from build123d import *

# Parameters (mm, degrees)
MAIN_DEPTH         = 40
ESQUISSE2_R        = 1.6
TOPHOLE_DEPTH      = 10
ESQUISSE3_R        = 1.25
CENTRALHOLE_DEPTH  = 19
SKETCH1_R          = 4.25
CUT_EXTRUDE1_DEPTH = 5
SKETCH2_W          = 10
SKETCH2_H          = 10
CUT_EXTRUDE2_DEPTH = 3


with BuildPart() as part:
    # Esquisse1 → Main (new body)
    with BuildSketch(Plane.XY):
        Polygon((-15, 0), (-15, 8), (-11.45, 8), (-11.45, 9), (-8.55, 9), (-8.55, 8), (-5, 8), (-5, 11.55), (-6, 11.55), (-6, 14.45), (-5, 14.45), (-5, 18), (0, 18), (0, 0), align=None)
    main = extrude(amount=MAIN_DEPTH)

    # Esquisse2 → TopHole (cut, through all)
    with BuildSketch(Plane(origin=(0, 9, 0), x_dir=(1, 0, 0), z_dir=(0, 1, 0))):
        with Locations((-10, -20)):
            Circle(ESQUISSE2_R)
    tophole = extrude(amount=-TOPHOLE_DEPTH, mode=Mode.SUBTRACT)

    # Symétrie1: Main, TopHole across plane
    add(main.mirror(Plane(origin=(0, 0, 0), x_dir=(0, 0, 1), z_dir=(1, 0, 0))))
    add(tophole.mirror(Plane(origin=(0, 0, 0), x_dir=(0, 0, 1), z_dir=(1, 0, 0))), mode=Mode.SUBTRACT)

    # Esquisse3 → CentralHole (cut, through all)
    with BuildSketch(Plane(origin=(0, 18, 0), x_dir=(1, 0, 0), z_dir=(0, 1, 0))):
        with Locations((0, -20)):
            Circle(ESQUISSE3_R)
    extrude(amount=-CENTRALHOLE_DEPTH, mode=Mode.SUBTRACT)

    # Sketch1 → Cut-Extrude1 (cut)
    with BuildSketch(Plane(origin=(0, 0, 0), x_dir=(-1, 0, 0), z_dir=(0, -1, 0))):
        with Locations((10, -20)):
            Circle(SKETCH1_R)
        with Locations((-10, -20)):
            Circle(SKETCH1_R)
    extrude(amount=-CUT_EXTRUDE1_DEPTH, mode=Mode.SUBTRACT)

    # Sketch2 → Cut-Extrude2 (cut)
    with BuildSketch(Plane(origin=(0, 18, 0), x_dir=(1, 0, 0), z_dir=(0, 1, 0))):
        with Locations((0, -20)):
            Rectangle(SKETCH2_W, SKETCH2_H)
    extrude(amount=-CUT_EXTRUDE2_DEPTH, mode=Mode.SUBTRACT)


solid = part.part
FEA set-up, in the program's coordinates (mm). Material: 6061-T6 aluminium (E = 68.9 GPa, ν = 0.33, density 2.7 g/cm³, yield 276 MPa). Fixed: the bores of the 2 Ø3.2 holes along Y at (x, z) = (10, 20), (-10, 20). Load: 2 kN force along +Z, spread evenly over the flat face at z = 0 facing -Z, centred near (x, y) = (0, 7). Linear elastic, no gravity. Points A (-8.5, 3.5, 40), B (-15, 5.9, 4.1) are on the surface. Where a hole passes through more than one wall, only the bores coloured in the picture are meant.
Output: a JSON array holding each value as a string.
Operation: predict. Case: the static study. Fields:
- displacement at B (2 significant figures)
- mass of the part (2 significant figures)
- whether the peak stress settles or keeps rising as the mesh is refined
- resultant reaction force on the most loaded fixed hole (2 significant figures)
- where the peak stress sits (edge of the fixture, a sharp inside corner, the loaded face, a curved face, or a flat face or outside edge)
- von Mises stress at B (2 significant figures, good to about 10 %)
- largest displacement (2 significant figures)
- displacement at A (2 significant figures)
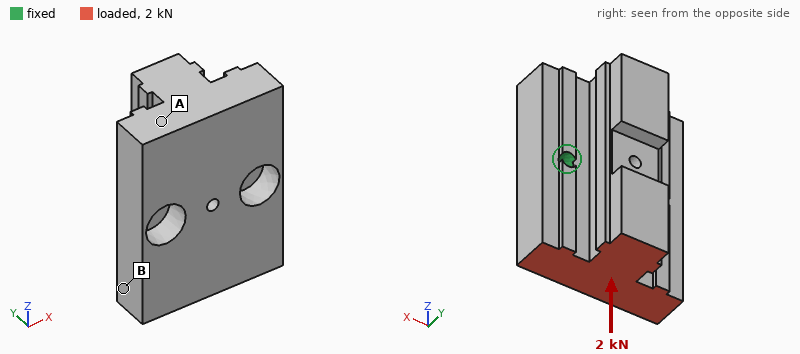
["3.0 µm", "35 g", "keeps rising", "1.0 kN", "edge of the fixture", "6.2 MPa", "4.2 µm", "1.5 µm"]
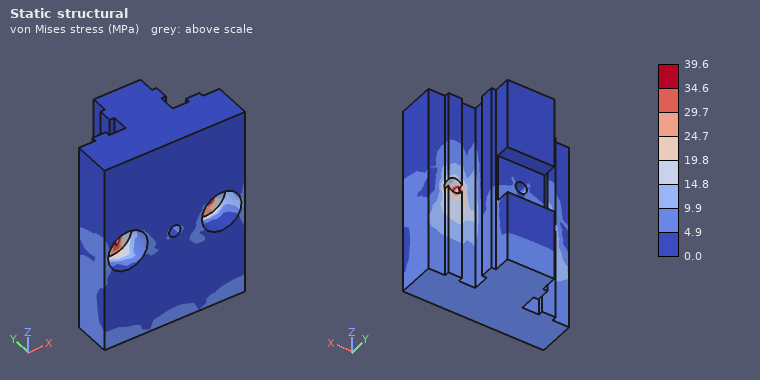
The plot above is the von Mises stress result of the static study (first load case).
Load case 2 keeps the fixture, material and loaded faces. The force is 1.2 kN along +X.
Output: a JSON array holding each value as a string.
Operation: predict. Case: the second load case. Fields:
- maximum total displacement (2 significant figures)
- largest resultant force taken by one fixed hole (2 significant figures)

["16 µm", "1.3 kN"]
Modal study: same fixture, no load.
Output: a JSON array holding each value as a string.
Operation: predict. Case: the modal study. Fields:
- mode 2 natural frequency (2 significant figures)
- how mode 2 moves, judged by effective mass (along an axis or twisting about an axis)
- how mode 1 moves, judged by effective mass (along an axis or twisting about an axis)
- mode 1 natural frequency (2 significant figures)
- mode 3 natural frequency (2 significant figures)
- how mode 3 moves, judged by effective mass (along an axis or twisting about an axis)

["13 kHz", "along Y", "twisting about X", "4500 Hz", "16 kHz", "twisting about Y"]
